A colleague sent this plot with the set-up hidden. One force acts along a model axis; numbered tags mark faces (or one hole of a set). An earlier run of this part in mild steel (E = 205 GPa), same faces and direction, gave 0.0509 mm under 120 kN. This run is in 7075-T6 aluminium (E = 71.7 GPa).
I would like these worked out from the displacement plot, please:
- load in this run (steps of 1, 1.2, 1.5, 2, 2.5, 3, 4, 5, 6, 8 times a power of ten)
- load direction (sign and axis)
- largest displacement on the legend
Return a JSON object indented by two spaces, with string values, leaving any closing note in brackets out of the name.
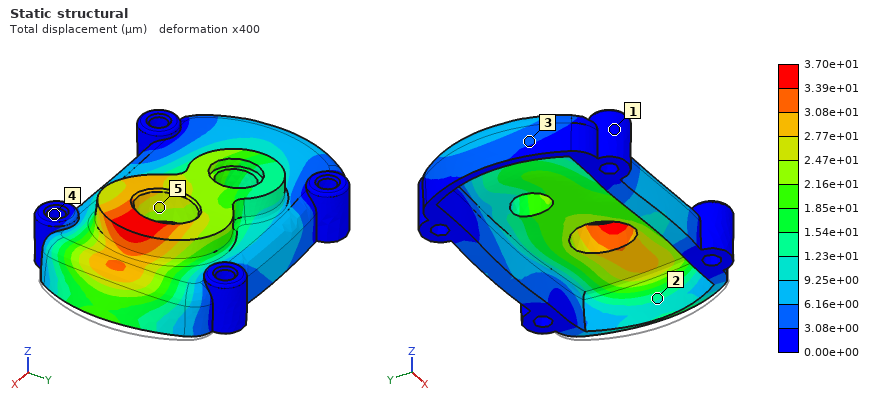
{
  "load in this run": "30 kN",
  "load direction": "-X",
  "largest displacement on the legend": "3.70e+01 µm"
}
